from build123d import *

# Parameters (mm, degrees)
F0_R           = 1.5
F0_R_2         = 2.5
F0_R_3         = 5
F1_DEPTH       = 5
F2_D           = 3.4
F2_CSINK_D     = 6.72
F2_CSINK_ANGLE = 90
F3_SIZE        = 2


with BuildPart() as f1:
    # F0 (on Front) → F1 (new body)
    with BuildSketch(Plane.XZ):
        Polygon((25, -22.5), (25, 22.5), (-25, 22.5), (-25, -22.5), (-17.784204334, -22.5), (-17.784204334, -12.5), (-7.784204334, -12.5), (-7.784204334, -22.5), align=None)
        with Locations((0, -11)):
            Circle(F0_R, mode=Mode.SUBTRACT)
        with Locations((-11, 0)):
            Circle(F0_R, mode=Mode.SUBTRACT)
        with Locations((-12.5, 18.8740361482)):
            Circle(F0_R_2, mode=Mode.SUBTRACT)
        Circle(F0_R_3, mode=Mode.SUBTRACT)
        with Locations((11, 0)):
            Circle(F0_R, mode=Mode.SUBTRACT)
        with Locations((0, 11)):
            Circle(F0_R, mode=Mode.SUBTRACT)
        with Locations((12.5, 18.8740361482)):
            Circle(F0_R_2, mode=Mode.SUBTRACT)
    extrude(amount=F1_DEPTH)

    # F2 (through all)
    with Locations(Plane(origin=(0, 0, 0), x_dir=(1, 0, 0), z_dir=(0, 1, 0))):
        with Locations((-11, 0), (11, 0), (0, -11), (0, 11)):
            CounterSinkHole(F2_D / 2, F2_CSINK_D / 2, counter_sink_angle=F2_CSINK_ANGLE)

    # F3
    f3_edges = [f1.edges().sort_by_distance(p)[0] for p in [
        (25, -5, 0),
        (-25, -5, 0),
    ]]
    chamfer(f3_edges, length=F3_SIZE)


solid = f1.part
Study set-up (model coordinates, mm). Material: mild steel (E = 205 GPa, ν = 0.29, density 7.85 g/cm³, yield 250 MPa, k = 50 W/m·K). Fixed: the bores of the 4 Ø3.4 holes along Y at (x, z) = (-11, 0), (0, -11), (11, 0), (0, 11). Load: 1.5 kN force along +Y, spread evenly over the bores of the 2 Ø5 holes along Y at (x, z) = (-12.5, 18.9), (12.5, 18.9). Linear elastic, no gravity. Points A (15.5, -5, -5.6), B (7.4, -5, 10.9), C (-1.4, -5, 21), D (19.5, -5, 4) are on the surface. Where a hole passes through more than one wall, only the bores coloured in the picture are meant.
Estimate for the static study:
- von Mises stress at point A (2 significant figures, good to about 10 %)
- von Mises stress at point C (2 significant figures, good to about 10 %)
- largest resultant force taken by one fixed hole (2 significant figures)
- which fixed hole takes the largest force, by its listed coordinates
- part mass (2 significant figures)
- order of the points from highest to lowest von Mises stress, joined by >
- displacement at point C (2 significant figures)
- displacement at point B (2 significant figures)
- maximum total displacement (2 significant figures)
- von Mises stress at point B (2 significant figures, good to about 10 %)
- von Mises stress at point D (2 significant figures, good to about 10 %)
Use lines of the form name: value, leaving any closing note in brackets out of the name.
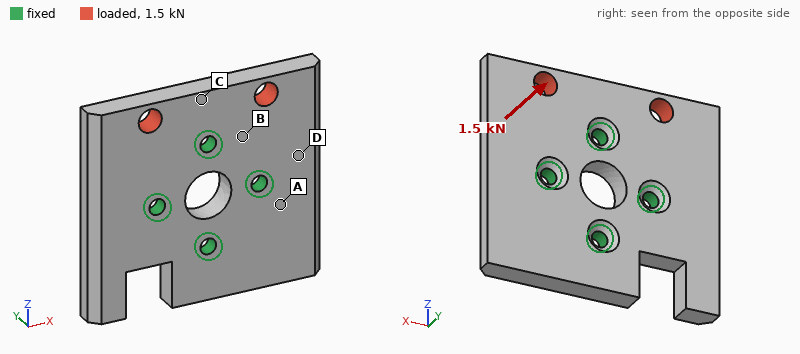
von Mises stress at point A: 17 MPa
von Mises stress at point C: 73 MPa
largest resultant force taken by one fixed hole: 1.5 kN
which fixed hole takes the largest force, by its listed coordinates: (0, 11)
part mass: 76 g
order of the points from highest to lowest von Mises stress, joined by >: C > B > D > A
displacement at point C: 12 µm
displacement at point B: 4.7 µm
maximum total displacement: 30 µm
von Mises stress at point B: 48 MPa
von Mises stress at point D: 36 MPa
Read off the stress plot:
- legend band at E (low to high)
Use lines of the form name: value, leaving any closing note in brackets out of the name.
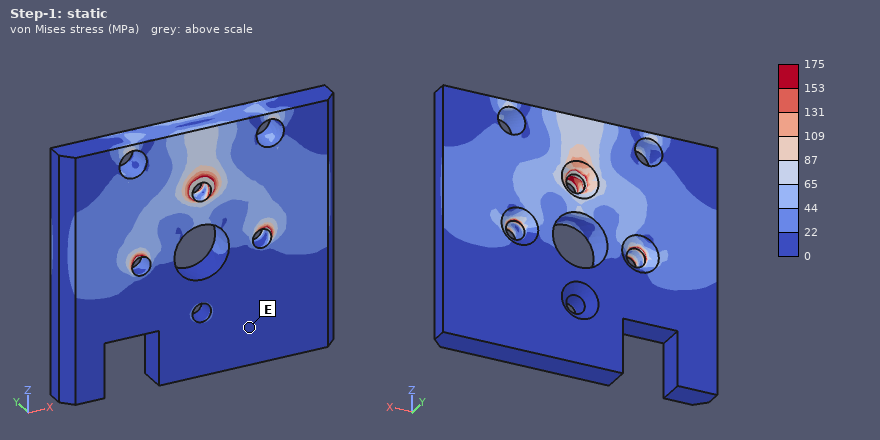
legend band at E: 0 to 22 MPa
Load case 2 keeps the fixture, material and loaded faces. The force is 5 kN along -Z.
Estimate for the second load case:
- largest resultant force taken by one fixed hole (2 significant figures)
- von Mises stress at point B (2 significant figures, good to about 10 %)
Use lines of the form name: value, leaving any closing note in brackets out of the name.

largest resultant force taken by one fixed hole: 1.6 kN
von Mises stress at point B: 23 MPa
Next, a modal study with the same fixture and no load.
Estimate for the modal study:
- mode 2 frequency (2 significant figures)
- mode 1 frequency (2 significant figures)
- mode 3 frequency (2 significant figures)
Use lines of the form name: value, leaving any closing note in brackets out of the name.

mode 2 frequency: 9100 Hz
mode 1 frequency: 8400 Hz
mode 3 frequency: 9400 Hz
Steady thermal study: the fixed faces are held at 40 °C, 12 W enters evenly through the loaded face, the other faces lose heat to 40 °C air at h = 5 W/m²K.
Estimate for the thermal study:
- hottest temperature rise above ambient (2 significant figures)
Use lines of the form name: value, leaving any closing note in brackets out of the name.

hottest temperature rise above ambient: 23 K
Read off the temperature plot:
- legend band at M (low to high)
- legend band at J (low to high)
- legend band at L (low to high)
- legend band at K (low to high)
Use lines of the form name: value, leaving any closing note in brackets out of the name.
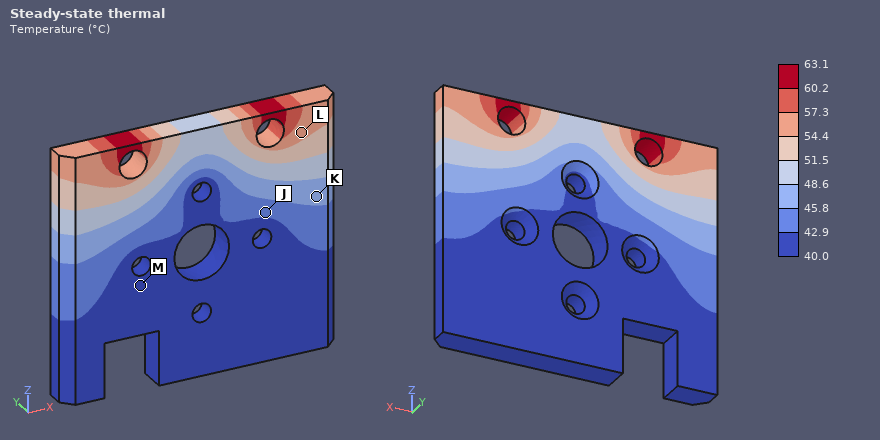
legend band at M: 40.0 to 42.9 °C
legend band at J: 42.9 to 45.8 °C
legend band at L: 54.4 to 57.3 °C
legend band at K: 45.8 to 48.6 °C
